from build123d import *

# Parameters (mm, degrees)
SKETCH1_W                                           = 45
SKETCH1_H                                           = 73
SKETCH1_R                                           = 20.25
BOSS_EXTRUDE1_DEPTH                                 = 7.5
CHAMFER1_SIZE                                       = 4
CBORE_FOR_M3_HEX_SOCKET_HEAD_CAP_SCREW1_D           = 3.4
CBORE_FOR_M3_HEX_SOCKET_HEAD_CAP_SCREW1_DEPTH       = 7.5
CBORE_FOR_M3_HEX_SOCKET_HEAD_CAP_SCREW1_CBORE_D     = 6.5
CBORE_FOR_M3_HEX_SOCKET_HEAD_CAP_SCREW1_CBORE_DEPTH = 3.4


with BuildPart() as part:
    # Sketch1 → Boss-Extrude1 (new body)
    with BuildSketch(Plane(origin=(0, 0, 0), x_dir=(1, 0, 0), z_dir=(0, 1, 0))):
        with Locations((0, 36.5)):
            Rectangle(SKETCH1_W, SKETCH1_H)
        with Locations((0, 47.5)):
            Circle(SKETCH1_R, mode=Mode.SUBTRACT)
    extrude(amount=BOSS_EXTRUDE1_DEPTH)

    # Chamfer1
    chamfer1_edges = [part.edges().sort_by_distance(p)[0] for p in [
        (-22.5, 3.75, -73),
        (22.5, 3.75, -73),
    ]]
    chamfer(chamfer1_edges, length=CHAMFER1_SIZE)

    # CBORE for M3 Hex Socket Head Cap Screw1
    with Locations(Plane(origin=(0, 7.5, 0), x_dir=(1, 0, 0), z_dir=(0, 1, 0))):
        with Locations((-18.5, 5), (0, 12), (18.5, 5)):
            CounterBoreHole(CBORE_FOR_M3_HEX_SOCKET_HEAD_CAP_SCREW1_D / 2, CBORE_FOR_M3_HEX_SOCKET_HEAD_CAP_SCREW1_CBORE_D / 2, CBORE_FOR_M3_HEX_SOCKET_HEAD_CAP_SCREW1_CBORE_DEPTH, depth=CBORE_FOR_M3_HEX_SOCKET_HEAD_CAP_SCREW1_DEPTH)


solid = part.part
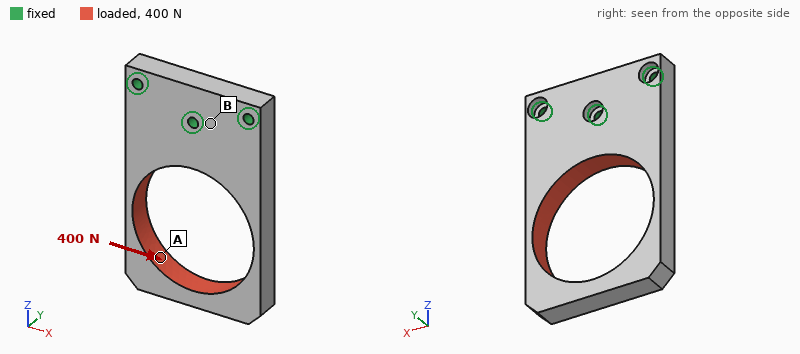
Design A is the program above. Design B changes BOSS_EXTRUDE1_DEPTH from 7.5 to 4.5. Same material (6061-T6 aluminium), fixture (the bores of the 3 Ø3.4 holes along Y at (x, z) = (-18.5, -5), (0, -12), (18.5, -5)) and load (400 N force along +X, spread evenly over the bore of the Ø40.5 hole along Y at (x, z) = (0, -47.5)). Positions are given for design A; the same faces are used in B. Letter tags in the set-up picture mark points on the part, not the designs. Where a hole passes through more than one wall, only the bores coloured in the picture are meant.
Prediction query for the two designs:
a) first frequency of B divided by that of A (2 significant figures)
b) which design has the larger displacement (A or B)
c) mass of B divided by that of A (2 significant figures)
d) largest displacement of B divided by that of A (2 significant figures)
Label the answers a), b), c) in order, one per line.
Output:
a) 0.66
b) B
c) 0.61
d) 1.6
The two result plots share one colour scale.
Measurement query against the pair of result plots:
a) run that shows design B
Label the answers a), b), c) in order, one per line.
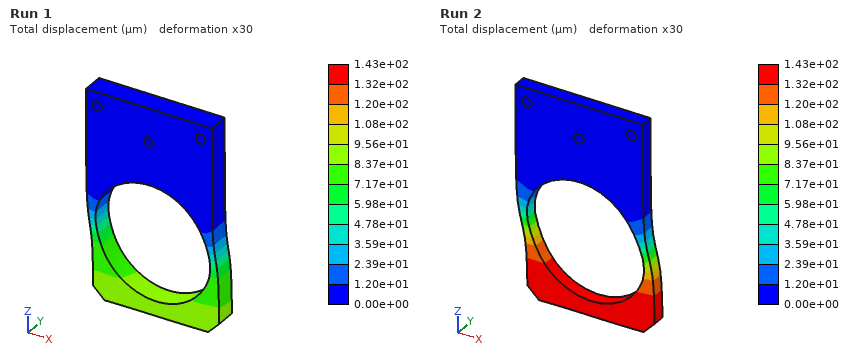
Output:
a) Run 2
